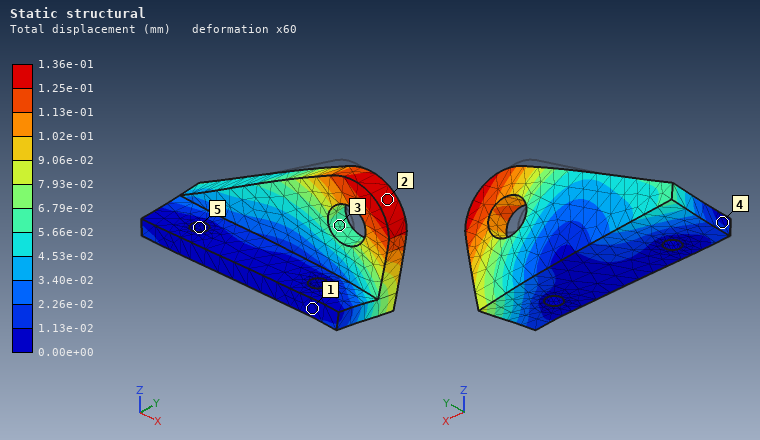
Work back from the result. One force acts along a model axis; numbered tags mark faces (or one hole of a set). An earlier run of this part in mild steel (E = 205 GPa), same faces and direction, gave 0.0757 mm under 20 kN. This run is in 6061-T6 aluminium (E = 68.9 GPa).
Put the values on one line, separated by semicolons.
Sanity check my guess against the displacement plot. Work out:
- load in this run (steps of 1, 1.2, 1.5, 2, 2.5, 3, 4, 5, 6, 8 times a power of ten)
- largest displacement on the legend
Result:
12 kN; 1.36e-01 mm
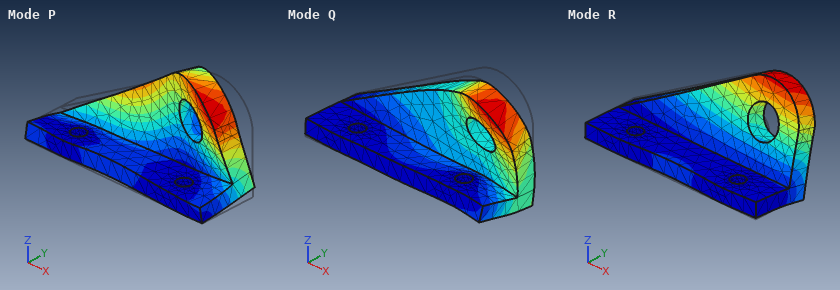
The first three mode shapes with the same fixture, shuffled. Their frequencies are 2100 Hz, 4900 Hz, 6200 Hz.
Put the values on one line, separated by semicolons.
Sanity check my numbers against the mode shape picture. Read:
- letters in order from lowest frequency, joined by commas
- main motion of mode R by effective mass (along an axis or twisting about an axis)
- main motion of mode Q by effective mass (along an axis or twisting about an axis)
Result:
R, P, Q; along Y; along Z
